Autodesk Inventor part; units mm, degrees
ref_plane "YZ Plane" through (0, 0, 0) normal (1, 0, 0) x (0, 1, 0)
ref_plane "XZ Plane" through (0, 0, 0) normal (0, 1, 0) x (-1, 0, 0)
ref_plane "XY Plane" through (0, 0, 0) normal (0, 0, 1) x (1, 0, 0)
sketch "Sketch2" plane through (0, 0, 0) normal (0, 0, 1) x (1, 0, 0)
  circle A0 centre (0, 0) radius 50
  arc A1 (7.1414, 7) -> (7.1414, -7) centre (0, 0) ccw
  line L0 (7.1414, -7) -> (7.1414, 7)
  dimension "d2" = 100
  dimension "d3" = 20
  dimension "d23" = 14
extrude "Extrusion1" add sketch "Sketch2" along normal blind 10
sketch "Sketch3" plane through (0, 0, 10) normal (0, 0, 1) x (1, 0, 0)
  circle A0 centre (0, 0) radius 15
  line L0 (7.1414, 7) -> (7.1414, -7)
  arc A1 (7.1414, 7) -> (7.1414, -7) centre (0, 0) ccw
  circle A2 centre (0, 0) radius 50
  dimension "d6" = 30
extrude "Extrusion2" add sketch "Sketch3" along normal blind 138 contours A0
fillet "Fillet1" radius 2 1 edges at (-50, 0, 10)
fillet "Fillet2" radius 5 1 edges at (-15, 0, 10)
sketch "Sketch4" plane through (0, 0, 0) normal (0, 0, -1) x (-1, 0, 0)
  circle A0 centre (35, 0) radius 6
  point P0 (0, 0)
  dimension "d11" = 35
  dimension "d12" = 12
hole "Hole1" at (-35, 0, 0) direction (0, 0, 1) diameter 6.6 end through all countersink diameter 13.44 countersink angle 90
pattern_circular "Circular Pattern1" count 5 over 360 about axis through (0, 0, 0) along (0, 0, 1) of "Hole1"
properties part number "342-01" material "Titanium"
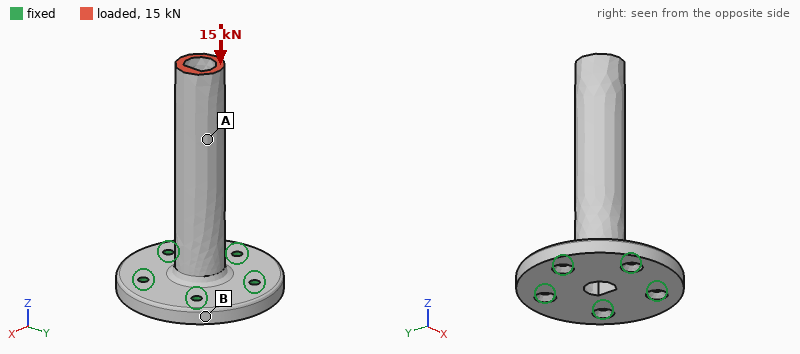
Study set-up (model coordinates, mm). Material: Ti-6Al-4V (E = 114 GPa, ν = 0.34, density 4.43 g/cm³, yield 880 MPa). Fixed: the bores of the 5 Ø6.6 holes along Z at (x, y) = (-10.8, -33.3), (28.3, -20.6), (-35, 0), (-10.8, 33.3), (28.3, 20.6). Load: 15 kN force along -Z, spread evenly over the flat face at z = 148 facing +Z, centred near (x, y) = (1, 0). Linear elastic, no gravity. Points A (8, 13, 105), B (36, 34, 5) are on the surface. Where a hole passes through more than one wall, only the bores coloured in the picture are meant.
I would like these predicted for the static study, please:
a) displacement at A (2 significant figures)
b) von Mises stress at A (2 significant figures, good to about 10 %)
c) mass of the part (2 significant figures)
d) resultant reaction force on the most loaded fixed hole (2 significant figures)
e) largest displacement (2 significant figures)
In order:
53 µm
35 MPa
580 g
3.1 kN
67 µm
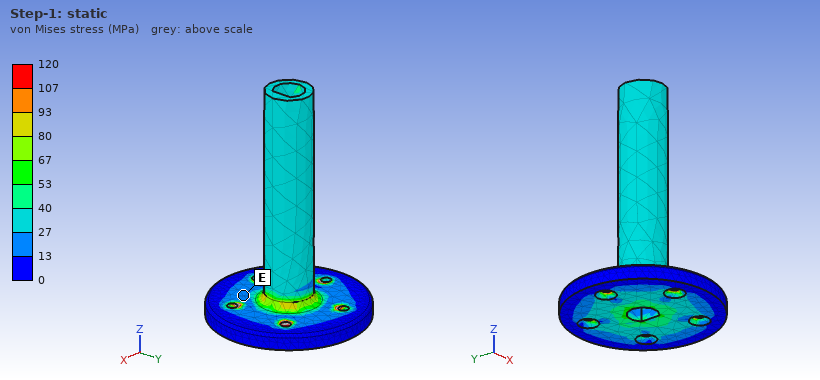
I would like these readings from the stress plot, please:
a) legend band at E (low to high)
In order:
13 to 27 MPa
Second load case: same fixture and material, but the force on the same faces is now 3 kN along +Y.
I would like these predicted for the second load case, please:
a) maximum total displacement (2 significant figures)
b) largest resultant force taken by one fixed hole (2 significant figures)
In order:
1.0 mm
5.2 kN
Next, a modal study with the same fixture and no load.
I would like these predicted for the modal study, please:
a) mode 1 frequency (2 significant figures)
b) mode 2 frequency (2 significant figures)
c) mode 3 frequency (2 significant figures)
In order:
1000 Hz
1000 Hz
5500 Hz
